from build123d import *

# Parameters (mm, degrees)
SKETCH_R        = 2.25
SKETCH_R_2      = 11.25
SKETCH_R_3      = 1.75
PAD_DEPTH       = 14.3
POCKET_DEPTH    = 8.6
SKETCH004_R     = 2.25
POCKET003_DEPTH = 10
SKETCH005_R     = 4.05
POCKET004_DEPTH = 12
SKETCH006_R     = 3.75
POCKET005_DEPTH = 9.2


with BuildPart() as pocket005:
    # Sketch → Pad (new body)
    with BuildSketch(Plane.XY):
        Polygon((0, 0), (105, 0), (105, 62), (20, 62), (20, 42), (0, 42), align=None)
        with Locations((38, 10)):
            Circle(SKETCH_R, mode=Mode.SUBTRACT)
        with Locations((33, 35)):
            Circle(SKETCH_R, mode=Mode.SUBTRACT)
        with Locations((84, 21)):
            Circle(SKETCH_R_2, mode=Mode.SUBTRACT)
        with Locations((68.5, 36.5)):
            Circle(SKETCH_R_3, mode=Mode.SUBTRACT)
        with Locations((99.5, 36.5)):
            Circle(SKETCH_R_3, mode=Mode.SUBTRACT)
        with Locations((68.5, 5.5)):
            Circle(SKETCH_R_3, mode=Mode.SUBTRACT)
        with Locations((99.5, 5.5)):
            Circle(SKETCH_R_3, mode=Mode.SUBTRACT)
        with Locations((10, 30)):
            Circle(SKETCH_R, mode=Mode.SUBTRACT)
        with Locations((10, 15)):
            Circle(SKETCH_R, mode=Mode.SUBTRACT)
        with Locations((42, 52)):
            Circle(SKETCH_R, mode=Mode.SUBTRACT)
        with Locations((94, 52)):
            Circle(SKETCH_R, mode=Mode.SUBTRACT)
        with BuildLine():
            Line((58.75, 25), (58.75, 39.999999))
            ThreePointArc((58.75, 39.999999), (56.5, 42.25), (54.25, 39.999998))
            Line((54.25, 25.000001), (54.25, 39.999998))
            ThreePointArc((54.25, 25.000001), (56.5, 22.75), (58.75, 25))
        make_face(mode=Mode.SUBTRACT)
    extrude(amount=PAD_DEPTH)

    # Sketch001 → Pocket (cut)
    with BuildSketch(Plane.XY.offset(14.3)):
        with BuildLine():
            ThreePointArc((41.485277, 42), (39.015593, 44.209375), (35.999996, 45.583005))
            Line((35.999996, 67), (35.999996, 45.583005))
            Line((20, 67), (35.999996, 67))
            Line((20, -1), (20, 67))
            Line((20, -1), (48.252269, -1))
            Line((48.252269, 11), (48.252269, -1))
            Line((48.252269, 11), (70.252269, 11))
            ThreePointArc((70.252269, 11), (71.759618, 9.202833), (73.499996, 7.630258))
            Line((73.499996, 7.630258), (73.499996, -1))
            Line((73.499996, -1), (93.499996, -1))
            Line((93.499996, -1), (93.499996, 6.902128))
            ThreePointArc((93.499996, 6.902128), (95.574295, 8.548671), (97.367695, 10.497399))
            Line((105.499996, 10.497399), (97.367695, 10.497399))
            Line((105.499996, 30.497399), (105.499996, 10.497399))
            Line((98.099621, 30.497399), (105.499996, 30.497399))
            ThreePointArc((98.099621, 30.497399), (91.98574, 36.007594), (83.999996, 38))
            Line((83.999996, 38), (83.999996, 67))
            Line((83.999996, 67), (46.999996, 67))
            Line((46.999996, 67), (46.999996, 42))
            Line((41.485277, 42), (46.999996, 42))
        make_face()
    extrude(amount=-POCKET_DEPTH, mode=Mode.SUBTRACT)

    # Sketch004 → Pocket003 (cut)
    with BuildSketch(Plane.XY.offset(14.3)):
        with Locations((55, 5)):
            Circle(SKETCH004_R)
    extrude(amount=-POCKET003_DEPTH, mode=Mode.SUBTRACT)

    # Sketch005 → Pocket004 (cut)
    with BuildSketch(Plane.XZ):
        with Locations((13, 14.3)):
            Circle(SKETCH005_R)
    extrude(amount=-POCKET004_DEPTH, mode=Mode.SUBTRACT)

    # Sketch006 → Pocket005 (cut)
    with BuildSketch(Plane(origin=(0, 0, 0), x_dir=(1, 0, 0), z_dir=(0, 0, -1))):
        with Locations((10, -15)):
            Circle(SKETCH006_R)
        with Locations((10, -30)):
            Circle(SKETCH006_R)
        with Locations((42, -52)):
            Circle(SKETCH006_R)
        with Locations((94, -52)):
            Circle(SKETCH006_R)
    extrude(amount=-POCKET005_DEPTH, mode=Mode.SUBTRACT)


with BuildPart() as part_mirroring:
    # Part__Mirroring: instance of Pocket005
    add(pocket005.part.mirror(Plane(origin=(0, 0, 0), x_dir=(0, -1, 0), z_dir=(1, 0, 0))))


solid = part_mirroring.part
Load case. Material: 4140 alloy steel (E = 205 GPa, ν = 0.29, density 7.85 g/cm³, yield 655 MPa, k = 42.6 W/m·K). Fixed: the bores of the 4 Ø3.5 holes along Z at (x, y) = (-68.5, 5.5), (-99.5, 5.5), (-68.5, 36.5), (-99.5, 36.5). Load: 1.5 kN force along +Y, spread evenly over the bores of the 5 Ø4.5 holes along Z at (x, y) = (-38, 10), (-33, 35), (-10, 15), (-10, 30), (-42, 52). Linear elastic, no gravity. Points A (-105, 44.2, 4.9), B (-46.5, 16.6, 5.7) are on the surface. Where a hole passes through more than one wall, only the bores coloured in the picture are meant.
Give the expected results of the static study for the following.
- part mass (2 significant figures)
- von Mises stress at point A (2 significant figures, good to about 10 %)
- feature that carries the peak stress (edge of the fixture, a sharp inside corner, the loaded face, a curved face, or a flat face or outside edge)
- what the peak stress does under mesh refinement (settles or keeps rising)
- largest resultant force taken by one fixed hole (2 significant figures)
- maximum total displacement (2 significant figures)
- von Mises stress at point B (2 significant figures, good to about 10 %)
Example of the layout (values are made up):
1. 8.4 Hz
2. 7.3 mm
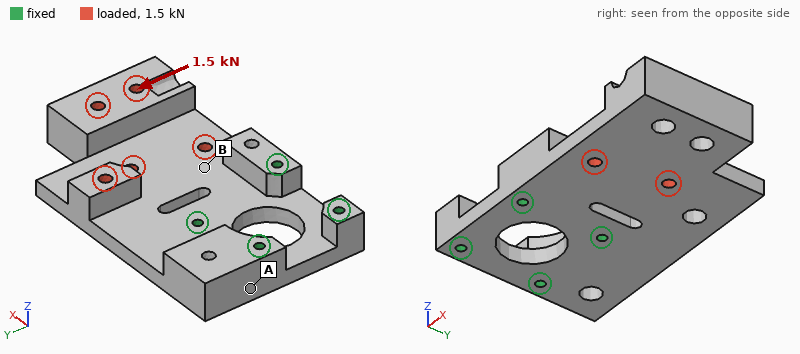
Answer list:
1. 360 g
2. 4.3 MPa
3. edge of the fixture
4. keeps rising
5. 1.5 kN
6. 30 µm
7. 25 MPa
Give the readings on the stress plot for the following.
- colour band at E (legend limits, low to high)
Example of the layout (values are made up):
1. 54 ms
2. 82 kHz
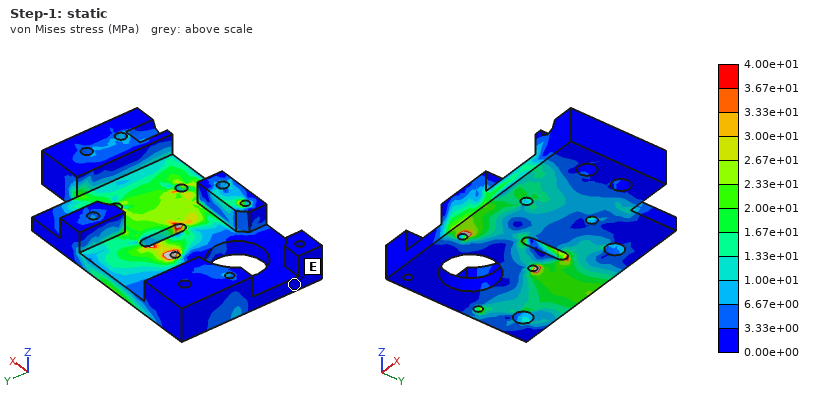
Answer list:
1. 0.00e+00 to 3.33e+00 MPa
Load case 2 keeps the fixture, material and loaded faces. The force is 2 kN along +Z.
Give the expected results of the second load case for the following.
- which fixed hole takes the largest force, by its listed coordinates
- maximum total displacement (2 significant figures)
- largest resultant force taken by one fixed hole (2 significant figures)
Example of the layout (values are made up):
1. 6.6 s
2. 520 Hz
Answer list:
1. (-68.5, 36.5)
2. 0.47 mm
3. 1.5 kN
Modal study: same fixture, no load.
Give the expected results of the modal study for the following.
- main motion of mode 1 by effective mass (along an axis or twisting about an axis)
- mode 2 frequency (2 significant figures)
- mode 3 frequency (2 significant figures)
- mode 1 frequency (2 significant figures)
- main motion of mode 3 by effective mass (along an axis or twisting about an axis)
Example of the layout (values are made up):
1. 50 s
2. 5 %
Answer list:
1. along Z
2. 2500 Hz
3. 4700 Hz
4. 920 Hz
5. along Y
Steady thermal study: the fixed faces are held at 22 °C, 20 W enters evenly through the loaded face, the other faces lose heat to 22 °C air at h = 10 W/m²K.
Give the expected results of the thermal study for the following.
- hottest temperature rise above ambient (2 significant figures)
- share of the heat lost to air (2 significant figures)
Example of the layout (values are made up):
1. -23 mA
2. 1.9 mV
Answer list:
1. 59 K
2. 22 %
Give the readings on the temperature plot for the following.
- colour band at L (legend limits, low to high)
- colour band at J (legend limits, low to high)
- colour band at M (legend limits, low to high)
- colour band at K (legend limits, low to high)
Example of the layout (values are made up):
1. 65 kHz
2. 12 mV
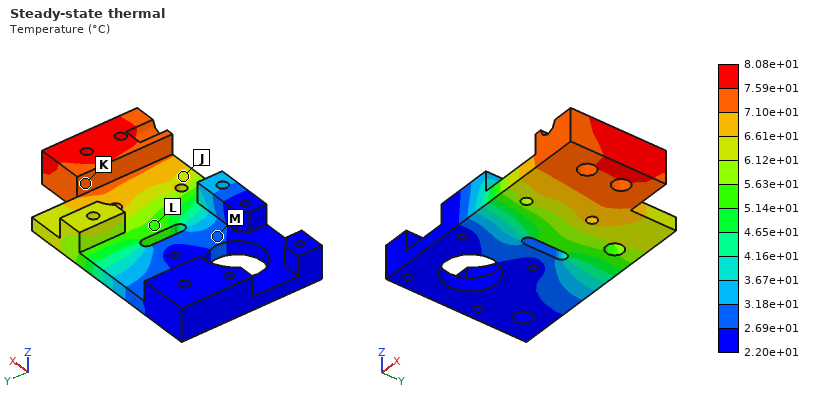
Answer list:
1. 5.14e+01 to 5.63e+01 °C
2. 6.12e+01 to 6.61e+01 °C
3. 2.69e+01 to 3.18e+01 °C
4. 7.10e+01 to 7.59e+01 °C
